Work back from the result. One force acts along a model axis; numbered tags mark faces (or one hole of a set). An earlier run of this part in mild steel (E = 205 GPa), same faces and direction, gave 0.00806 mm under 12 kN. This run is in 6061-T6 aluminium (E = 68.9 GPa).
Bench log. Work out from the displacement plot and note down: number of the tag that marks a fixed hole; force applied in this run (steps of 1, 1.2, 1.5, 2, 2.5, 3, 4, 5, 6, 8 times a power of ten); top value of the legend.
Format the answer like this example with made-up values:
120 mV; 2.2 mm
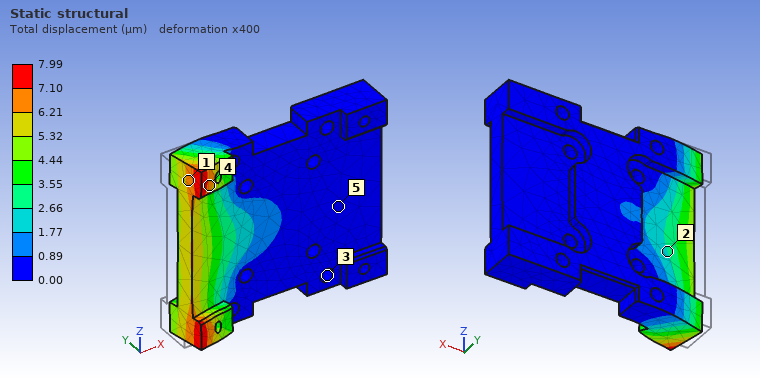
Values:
3; 4 kN; 7.99 µm
